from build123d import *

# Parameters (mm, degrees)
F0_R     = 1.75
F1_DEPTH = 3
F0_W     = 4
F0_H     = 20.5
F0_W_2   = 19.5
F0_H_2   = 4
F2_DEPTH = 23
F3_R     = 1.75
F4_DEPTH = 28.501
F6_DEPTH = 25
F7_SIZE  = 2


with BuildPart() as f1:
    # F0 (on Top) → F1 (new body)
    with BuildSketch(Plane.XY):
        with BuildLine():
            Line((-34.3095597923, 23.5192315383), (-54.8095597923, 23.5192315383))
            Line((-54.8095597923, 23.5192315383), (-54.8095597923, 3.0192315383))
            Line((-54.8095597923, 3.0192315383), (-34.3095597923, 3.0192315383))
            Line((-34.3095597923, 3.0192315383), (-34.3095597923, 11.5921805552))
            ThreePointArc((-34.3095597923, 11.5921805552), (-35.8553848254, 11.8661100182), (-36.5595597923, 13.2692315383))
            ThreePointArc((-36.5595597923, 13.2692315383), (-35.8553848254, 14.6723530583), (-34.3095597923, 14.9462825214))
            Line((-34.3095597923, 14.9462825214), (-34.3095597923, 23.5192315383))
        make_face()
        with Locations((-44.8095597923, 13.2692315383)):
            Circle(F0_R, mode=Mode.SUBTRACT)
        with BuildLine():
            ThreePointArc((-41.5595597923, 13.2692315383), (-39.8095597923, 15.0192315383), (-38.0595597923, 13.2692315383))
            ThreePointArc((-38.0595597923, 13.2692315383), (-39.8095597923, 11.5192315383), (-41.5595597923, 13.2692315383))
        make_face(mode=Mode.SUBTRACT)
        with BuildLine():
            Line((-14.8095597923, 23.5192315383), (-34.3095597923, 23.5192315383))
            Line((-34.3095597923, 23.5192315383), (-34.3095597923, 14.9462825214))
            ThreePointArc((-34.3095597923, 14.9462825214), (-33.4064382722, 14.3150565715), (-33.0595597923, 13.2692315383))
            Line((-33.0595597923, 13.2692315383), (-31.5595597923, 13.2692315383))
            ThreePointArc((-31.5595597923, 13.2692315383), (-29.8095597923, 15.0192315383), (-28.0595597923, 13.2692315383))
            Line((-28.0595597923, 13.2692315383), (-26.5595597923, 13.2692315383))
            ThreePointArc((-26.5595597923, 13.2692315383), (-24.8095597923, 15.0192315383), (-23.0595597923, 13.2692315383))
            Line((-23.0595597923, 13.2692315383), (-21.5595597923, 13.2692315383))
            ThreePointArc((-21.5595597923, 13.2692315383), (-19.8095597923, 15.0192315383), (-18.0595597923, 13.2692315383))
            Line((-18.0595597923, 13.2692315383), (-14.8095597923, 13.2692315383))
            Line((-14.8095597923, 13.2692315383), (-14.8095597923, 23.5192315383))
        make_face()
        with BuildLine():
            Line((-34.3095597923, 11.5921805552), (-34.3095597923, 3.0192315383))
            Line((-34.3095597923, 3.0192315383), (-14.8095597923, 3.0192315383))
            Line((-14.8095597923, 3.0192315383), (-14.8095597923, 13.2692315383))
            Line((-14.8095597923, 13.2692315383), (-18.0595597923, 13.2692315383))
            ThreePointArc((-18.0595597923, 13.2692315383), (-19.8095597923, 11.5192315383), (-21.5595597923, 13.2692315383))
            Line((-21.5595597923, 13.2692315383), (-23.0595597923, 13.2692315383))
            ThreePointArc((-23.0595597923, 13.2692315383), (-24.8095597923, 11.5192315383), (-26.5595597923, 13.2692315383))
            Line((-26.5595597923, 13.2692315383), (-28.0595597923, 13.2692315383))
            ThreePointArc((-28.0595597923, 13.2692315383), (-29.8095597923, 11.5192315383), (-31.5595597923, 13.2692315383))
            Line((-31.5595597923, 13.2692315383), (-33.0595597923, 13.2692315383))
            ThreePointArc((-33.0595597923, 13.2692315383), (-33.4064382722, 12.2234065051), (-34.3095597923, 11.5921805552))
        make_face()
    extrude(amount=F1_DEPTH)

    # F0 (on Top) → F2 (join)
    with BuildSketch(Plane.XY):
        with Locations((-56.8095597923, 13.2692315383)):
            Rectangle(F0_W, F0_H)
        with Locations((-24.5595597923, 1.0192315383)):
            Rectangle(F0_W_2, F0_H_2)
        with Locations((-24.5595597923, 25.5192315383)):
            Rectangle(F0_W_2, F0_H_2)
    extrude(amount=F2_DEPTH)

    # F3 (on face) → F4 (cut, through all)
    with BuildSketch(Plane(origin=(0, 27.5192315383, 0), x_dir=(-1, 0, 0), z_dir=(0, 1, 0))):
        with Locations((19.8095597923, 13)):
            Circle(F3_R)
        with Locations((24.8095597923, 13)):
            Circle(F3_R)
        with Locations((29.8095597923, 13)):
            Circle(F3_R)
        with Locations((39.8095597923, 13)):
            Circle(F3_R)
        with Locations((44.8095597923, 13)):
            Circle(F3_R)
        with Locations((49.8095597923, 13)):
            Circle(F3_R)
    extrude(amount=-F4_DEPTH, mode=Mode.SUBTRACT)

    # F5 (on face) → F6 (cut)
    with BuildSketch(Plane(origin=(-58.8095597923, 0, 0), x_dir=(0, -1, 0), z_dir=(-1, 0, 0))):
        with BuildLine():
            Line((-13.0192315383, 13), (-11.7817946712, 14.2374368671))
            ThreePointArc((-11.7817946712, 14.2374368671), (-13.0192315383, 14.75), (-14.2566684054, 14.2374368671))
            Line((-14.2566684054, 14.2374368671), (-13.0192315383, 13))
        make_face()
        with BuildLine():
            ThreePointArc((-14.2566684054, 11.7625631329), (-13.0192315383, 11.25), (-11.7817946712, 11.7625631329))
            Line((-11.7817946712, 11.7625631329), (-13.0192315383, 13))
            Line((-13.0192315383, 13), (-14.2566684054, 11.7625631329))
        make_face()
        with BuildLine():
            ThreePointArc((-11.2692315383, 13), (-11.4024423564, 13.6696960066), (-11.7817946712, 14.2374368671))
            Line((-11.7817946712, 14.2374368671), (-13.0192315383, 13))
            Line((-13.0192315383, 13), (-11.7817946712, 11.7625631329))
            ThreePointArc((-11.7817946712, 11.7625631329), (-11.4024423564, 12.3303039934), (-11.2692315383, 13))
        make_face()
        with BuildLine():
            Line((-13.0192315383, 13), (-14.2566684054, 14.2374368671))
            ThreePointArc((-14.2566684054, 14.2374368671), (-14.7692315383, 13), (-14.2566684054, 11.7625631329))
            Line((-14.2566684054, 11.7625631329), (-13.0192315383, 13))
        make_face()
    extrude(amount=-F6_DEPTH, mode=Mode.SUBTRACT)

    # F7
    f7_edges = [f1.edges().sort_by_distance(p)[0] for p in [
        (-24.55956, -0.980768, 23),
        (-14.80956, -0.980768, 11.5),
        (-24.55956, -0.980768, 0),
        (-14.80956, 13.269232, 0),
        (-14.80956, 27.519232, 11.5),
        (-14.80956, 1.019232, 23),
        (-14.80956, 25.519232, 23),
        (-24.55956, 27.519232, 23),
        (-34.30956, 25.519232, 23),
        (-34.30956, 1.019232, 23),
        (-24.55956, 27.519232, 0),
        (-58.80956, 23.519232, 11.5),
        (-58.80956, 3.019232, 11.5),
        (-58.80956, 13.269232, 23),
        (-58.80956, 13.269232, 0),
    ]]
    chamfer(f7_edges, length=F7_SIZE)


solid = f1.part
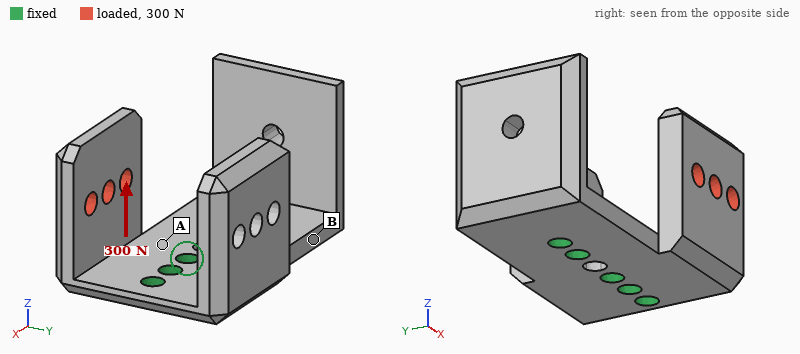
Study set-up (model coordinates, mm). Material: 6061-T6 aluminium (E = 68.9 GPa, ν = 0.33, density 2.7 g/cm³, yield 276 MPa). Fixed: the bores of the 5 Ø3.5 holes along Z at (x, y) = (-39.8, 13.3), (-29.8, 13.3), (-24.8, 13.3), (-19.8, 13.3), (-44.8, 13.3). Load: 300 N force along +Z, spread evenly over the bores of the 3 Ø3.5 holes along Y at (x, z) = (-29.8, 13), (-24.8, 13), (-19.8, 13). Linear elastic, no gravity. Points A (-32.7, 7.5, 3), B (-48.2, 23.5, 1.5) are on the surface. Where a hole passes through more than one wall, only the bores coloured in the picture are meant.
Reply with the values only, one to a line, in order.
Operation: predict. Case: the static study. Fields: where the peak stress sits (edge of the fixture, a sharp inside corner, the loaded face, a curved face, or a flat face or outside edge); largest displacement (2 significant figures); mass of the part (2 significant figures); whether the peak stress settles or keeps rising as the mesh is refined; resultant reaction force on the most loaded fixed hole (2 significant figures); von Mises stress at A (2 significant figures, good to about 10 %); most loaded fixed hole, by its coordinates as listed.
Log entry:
edge of the fixture
0.12 mm
19 g
keeps rising
110 N
44 MPa
(-19.8, 13.3)
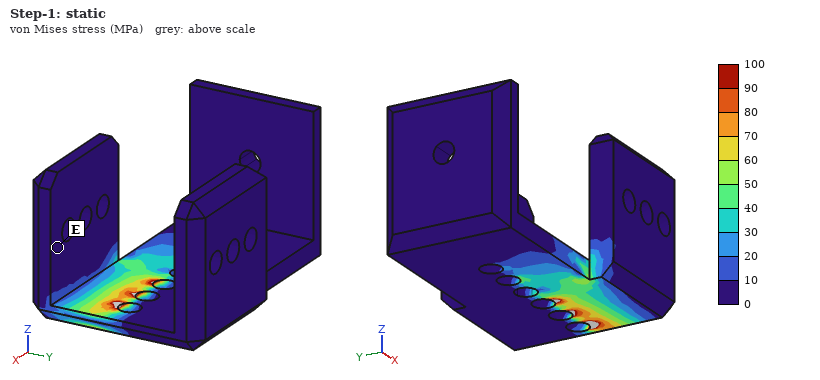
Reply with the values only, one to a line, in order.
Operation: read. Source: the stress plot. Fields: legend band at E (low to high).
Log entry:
0 to 10 MPa
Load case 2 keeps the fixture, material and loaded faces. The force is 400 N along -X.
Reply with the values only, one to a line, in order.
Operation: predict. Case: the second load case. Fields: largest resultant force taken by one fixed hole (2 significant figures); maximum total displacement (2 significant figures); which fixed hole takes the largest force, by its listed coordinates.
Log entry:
330 N
0.10 mm
(-19.8, 13.3)
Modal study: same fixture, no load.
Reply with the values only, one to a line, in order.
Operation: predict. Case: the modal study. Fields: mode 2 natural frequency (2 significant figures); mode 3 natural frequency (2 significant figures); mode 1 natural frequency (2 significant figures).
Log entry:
3200 Hz
3200 Hz
2800 Hz
